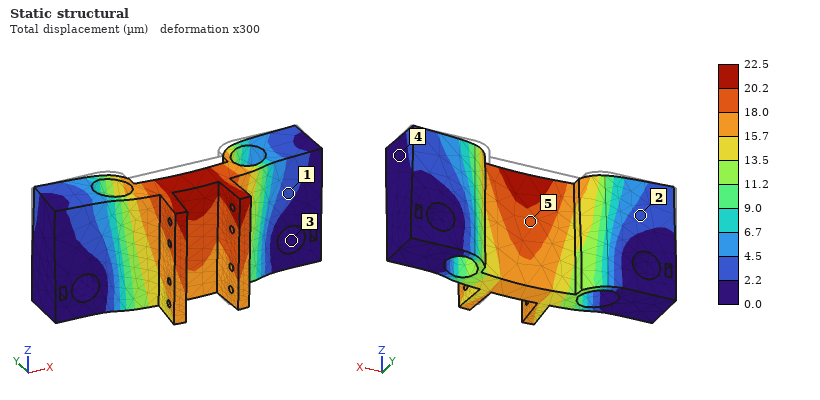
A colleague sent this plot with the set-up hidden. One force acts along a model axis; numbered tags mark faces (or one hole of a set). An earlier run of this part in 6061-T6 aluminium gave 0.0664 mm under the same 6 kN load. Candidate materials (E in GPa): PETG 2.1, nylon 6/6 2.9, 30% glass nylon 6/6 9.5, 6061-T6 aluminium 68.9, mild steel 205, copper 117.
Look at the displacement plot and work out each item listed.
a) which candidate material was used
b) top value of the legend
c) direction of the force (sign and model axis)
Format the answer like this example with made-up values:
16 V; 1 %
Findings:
mild steel; 22.5 µm; -Y
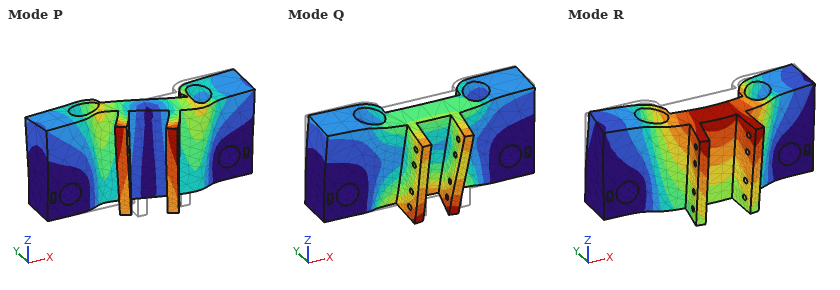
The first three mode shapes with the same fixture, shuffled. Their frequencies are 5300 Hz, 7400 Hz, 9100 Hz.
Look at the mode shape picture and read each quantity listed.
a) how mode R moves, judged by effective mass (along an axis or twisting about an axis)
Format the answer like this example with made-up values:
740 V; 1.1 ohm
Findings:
along Y
